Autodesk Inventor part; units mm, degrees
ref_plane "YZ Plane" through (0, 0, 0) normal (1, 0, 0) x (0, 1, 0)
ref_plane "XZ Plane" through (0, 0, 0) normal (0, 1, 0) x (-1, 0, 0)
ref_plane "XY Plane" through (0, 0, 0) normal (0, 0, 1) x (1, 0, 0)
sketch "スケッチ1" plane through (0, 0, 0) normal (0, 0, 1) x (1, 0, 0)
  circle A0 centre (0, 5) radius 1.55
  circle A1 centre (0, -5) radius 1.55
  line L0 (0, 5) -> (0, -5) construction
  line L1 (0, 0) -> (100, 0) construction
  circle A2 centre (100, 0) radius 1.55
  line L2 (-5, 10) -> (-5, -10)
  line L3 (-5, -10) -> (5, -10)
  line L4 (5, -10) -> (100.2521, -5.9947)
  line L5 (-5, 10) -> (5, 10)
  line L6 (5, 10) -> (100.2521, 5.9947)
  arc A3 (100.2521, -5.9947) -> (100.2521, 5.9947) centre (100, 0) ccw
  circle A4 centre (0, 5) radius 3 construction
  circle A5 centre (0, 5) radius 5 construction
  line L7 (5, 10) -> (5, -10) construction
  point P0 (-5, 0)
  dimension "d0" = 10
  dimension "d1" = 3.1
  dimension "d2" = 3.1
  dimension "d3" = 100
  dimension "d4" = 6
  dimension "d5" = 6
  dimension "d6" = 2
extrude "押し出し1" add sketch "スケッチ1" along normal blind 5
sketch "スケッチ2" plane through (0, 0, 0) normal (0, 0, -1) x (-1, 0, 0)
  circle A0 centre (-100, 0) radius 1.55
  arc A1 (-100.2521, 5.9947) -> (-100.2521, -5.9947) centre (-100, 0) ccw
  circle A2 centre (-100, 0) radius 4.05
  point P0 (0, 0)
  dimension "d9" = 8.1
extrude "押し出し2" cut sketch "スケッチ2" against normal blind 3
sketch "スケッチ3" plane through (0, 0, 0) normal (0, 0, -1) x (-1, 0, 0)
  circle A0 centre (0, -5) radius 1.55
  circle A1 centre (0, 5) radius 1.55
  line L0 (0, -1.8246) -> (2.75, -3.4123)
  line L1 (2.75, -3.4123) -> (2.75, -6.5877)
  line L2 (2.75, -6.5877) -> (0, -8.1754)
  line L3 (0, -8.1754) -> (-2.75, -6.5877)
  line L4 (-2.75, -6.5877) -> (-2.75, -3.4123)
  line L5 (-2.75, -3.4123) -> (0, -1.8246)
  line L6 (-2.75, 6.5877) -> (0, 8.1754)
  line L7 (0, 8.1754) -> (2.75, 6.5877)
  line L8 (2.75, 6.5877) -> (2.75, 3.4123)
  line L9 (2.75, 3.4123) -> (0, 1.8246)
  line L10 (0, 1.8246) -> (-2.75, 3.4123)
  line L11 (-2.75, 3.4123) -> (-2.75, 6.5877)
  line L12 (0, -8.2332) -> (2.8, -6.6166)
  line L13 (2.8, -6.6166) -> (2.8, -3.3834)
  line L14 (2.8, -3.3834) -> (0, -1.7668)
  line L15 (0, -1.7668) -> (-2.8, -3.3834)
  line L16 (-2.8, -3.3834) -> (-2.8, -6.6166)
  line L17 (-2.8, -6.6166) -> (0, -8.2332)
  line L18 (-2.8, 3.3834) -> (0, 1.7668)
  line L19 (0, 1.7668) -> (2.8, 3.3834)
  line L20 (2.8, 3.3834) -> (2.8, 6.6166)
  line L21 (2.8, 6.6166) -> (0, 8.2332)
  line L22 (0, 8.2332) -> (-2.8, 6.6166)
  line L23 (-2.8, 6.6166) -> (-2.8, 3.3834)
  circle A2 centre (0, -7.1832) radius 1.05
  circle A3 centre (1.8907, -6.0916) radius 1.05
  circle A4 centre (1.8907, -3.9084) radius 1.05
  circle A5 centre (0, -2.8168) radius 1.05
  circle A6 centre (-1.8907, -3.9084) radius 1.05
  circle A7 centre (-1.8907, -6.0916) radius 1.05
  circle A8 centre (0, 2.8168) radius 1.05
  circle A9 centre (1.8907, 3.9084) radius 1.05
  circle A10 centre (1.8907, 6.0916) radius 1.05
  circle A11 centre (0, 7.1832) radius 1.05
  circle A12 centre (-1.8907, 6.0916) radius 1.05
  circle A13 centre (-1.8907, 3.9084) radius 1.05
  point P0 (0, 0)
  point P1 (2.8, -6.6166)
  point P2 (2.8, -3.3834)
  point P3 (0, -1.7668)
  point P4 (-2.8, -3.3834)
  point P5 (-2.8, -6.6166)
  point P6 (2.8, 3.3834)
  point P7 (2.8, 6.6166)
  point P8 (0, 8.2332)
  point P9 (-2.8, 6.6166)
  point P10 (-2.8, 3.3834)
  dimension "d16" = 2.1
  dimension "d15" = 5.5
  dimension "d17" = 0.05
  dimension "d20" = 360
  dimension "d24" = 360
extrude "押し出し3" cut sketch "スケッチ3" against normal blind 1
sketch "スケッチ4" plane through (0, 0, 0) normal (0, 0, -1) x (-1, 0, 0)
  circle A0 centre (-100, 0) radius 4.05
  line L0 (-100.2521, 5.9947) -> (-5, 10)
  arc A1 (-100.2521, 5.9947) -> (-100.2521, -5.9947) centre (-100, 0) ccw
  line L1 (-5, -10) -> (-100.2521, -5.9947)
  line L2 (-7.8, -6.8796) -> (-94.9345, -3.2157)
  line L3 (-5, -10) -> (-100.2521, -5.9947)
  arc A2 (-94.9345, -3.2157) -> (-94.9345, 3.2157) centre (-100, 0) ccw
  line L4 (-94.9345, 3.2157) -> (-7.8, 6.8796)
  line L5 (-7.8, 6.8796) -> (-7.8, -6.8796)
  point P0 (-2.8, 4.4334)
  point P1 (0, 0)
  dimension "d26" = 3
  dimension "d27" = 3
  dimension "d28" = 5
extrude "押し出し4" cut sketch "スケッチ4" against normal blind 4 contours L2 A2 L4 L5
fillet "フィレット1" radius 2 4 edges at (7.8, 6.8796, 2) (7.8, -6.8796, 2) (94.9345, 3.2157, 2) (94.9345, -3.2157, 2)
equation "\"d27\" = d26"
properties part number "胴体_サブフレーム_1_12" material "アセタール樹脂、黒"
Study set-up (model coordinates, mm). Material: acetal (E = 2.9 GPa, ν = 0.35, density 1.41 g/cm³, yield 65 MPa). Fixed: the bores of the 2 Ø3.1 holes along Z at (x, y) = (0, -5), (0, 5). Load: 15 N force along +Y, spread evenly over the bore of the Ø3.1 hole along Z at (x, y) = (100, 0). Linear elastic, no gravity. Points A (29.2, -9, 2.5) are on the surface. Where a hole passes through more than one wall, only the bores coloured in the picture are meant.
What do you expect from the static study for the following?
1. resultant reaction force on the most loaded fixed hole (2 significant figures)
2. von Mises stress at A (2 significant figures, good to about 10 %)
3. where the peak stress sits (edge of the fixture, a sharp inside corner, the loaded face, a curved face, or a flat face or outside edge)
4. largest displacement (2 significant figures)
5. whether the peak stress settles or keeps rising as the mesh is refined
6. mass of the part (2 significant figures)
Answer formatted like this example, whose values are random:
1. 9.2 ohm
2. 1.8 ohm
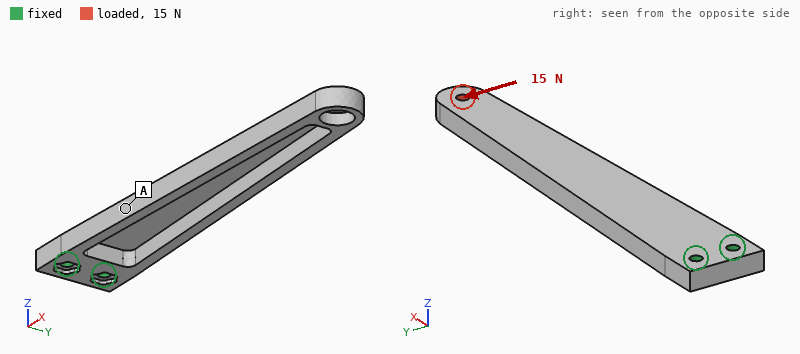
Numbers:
1. 120 N
2. 5.3 MPa
3. edge of the fixture
4. 1.2 mm
5. keeps rising
6. 7.2 g
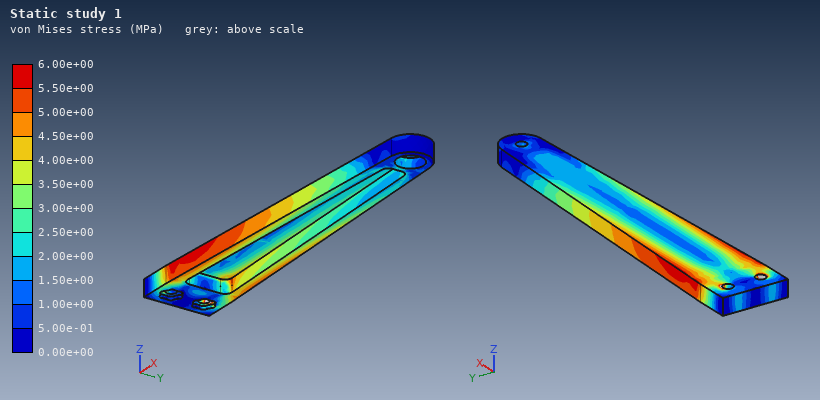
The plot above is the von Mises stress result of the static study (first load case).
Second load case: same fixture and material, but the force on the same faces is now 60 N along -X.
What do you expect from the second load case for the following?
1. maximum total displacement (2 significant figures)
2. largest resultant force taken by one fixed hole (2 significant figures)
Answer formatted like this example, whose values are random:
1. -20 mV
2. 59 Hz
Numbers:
1. 1.1 mm
2. 30 N
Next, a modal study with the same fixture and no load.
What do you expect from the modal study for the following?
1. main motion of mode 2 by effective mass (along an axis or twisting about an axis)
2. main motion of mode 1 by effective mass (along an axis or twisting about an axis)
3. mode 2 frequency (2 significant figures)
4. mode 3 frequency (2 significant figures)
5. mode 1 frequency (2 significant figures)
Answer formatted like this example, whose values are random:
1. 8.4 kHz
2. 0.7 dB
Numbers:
1. along Y
2. along Z
3. 430 Hz
4. 680 Hz
5. 120 Hz
